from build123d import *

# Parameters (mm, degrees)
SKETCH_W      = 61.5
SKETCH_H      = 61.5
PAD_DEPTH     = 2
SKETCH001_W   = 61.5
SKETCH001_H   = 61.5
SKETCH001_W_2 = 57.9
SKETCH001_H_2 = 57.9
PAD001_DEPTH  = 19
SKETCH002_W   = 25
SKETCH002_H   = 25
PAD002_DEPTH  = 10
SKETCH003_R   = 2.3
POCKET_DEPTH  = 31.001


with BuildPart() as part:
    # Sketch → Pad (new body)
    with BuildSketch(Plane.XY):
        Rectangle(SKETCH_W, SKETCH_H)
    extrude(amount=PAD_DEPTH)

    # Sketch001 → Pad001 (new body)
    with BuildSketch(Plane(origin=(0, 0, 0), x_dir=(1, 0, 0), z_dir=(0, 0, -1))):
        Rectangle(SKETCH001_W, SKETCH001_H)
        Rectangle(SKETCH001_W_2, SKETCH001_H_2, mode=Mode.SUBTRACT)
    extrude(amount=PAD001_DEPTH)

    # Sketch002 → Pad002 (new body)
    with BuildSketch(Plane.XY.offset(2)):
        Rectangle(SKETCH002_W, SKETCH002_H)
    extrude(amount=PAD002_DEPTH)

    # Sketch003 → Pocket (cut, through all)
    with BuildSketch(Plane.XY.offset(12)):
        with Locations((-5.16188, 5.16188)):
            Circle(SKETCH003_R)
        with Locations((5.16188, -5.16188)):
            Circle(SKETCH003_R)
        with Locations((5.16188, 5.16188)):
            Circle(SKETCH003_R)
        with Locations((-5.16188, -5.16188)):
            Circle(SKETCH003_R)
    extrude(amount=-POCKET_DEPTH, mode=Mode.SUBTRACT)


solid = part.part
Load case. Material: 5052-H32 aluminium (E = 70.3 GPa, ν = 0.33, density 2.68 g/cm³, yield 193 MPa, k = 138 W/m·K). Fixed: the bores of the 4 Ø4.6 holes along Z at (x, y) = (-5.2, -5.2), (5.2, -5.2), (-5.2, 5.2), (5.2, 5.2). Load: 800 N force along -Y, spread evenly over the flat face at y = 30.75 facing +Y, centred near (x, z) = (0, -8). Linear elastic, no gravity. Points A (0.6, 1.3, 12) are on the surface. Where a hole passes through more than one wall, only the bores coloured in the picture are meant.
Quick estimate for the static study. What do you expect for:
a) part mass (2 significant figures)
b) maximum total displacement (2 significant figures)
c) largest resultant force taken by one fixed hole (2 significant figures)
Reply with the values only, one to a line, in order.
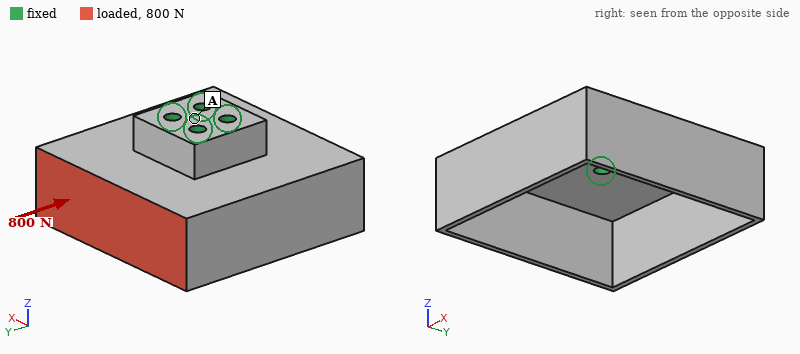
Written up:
57 g
0.44 mm
350 N
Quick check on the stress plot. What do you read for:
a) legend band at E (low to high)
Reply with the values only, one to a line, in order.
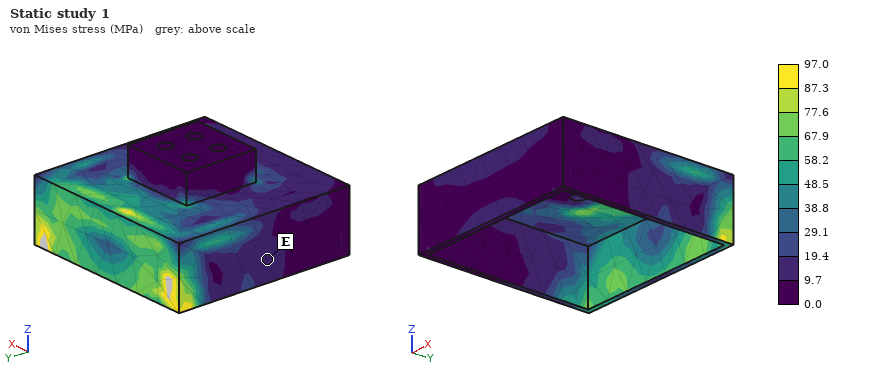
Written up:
9.7 to 19.4 MPa
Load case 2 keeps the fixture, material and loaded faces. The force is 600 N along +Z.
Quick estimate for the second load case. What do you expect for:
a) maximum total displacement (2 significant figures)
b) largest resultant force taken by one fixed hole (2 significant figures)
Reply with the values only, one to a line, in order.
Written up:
0.41 mm
490 N
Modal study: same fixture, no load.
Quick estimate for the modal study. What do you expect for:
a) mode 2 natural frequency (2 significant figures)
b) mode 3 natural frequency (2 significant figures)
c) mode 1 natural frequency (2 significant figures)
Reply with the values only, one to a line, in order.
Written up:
1800 Hz
1800 Hz
1600 Hz
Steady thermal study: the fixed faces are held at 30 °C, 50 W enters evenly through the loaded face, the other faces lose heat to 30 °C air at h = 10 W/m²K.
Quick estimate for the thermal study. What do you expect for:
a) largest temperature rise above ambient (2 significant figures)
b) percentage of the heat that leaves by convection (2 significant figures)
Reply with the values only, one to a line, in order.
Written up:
80 K
7.4 %
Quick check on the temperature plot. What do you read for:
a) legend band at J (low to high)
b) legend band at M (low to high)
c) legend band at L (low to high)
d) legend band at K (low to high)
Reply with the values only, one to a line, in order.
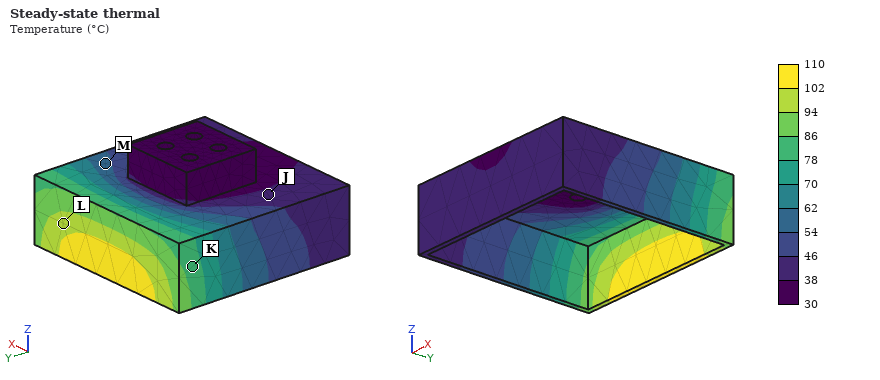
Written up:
38 to 46 °C
54 to 62 °C
94 to 102 °C
78 to 86 °C
